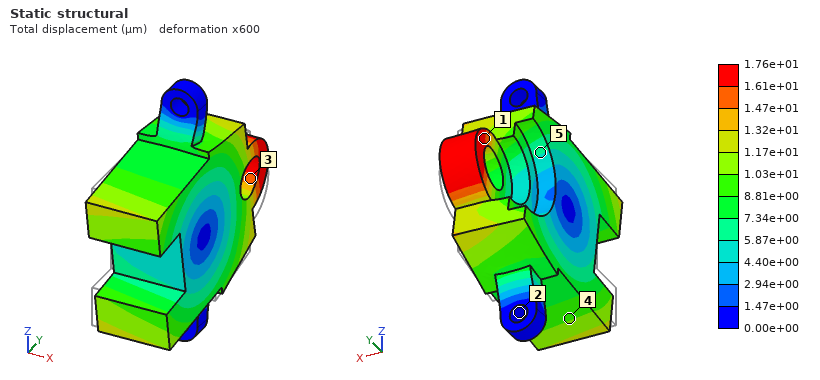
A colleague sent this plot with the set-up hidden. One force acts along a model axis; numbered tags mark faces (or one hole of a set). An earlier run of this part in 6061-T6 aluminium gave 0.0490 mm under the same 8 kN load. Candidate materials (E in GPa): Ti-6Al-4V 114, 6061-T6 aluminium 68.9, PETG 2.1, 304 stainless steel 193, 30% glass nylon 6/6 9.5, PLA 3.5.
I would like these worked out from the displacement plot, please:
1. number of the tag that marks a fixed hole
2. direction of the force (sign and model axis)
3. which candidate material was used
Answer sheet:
2
+Z
304 stainless steel
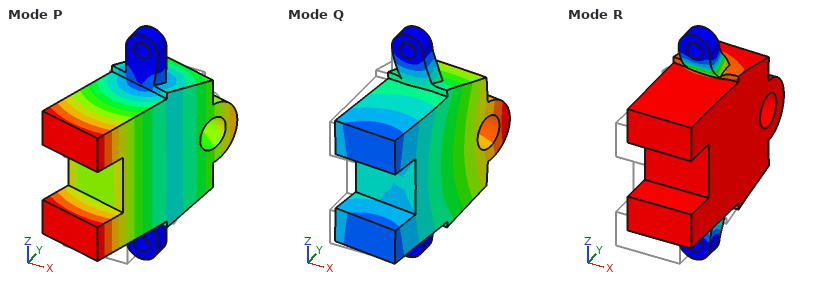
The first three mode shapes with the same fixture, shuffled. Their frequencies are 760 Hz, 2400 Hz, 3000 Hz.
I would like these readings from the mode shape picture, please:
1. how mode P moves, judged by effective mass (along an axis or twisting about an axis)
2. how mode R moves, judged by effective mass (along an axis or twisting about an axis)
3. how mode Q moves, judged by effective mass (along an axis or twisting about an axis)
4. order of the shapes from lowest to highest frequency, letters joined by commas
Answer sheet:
along X
along Y
along X
P, R, Q
